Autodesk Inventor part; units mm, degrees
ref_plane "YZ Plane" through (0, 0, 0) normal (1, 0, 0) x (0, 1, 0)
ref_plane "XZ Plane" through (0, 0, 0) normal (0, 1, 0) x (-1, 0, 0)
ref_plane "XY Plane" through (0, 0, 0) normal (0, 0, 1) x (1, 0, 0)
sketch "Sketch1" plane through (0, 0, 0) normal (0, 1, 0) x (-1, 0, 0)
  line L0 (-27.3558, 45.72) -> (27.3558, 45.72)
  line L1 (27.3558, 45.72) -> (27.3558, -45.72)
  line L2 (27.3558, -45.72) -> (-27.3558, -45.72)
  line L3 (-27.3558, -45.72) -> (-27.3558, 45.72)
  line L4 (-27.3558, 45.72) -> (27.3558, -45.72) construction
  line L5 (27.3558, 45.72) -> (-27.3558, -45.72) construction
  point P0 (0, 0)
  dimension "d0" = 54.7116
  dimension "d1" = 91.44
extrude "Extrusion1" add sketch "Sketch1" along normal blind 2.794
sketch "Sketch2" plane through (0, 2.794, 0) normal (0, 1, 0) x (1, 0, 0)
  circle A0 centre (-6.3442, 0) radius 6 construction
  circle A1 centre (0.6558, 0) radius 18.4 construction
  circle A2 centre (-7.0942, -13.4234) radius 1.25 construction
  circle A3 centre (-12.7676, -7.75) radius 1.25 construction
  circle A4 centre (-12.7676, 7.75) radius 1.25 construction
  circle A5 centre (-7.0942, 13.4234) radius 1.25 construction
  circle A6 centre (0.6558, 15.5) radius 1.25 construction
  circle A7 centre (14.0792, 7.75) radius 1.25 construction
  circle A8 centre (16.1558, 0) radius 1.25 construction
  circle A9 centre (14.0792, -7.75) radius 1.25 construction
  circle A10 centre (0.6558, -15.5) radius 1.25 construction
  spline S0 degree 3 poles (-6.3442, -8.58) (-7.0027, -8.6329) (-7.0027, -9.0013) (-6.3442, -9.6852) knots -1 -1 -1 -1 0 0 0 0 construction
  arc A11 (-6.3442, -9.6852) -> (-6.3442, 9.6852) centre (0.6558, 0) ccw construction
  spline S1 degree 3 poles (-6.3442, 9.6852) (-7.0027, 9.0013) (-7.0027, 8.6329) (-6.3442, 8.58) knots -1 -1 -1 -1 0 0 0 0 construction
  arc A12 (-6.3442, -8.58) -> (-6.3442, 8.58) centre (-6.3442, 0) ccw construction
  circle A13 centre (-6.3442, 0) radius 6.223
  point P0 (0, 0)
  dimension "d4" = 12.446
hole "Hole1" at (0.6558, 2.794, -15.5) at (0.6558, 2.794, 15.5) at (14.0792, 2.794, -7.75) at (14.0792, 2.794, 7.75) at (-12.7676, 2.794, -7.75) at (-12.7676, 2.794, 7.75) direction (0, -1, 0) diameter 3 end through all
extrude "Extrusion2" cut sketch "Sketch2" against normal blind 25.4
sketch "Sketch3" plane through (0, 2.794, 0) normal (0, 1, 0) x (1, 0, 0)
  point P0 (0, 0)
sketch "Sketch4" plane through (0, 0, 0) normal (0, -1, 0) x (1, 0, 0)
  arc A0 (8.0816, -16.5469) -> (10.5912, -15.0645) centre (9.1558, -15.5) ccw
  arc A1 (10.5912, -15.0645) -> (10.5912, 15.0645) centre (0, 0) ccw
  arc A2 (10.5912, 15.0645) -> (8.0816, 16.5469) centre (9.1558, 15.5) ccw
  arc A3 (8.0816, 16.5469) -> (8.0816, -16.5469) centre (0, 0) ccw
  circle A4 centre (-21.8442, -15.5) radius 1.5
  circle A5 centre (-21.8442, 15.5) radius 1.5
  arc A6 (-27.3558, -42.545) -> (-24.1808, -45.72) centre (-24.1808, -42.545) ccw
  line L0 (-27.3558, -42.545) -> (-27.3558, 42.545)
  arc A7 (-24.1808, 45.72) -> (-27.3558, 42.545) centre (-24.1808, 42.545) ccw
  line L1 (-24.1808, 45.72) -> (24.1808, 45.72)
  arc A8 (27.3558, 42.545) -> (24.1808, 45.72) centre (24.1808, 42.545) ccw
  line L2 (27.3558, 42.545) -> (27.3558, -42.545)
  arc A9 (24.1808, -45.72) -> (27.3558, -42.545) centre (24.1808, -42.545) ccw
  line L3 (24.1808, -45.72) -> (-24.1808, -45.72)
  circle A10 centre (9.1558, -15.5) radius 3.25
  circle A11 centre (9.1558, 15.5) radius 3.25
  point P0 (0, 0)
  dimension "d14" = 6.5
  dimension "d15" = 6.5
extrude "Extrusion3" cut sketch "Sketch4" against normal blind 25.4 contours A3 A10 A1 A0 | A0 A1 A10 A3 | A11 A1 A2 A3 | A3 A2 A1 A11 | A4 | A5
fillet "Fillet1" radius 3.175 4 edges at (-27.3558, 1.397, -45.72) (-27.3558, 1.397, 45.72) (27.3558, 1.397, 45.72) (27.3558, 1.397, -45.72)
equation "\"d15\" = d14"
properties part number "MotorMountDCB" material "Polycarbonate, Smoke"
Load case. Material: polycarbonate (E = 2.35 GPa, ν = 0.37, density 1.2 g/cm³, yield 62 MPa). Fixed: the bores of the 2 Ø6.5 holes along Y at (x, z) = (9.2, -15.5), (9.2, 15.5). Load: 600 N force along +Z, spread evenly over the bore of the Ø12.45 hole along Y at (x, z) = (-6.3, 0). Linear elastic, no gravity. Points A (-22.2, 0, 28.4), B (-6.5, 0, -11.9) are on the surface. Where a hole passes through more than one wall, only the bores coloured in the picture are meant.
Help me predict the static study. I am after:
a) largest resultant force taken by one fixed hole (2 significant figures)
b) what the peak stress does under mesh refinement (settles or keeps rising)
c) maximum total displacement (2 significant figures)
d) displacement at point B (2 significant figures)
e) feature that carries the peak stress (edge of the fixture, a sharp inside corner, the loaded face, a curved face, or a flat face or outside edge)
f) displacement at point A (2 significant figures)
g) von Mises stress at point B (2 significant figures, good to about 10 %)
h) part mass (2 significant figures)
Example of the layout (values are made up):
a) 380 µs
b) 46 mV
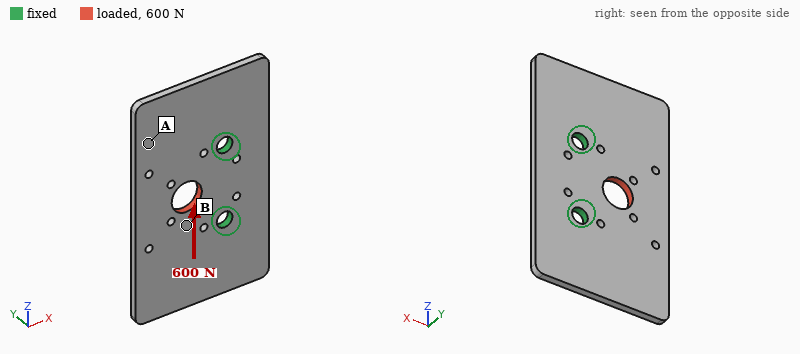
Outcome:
a) 380 N
b) keeps rising
c) 0.21 mm
d) 0.10 mm
e) edge of the fixture
f) 0.16 mm
g) 6.9 MPa
h) 16 g
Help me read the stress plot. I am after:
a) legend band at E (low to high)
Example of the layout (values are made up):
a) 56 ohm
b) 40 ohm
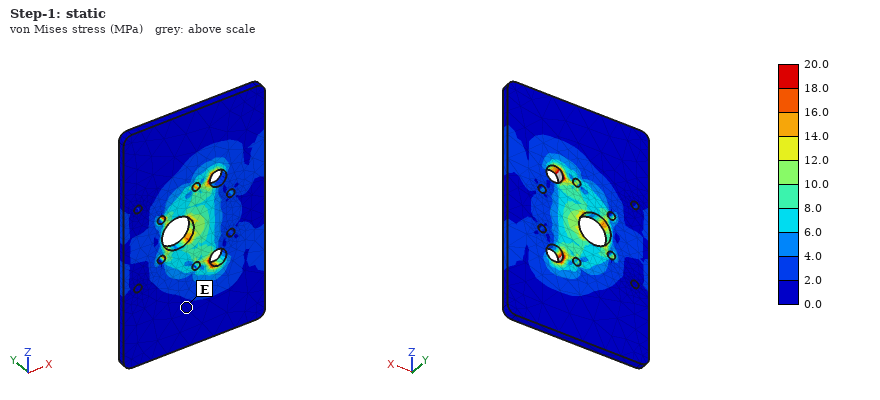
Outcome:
a) 0.0 to 2.0 MPa
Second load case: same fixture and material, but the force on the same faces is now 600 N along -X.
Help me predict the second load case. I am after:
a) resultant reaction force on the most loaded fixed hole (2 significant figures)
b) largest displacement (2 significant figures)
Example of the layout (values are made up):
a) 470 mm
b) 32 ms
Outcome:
a) 310 N
b) 83 µm
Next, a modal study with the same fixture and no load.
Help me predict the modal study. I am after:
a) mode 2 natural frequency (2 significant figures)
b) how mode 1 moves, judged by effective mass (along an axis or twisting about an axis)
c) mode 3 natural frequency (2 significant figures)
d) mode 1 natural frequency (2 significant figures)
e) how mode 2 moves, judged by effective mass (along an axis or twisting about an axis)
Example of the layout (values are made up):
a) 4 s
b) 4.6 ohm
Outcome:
a) 460 Hz
b) along Y
c) 680 Hz
d) 420 Hz
e) twisting about X
